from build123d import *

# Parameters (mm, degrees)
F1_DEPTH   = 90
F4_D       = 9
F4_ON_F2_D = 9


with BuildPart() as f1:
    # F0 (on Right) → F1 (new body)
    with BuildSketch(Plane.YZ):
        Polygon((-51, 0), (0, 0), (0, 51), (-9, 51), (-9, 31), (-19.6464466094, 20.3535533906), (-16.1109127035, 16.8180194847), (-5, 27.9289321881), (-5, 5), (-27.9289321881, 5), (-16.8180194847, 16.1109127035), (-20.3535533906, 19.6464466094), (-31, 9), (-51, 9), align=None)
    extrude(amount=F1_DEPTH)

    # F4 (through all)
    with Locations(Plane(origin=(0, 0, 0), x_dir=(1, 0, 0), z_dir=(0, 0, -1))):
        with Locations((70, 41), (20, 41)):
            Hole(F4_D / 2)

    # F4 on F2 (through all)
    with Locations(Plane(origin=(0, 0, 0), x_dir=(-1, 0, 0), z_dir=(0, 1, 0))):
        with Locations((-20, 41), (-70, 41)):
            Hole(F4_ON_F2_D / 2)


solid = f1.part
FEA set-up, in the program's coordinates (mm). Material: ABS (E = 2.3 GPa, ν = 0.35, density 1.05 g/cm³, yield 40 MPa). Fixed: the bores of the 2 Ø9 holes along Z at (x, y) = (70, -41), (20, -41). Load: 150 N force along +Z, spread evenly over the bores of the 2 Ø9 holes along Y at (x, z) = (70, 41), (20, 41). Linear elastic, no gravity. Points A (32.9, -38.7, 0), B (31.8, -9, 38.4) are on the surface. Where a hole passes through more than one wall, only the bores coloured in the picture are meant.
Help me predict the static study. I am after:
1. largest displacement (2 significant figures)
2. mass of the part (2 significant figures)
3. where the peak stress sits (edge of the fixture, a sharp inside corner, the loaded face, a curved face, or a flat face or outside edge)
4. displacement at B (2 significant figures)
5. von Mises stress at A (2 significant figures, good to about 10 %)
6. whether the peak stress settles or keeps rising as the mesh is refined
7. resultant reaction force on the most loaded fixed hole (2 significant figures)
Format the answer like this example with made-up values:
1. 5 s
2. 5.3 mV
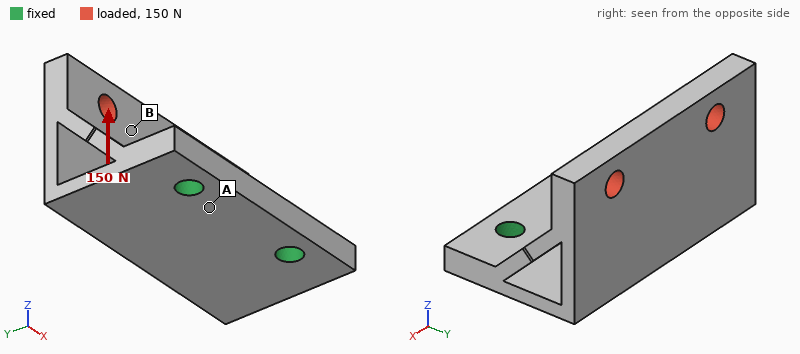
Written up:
1. 1.2 mm
2. 74 g
3. edge of the fixture
4. 0.89 mm
5. 2.1 MPa
6. keeps rising
7. 75 N
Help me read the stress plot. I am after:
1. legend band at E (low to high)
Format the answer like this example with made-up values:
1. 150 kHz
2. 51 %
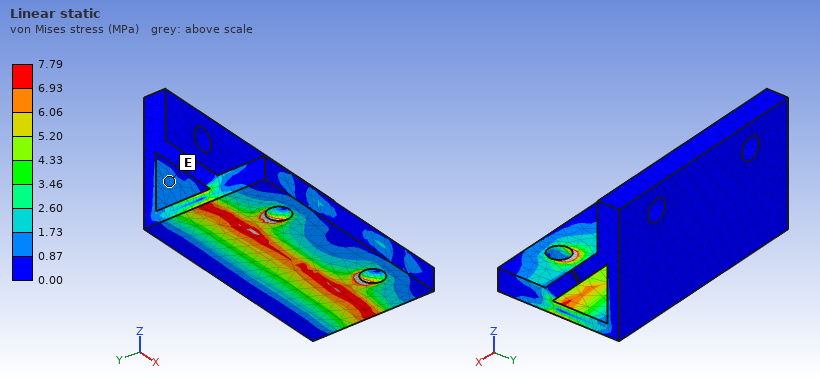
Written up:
1. 0.87 to 1.73 MPa
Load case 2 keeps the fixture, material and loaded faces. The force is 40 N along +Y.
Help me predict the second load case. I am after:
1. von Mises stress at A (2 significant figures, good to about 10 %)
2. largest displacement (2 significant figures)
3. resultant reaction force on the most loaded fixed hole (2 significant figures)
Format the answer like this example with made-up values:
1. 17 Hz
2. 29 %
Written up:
1. 0.62 MPa
2. 1.3 mm
3. 20 N
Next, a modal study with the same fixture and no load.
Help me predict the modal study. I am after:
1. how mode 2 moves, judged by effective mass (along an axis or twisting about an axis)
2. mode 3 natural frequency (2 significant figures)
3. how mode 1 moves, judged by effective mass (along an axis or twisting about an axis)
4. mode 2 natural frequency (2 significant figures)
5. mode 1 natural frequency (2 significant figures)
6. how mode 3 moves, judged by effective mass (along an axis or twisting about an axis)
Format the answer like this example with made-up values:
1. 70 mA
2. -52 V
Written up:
1. along X
2. 570 Hz
3. along Y
4. 390 Hz
5. 210 Hz
6. along Z
